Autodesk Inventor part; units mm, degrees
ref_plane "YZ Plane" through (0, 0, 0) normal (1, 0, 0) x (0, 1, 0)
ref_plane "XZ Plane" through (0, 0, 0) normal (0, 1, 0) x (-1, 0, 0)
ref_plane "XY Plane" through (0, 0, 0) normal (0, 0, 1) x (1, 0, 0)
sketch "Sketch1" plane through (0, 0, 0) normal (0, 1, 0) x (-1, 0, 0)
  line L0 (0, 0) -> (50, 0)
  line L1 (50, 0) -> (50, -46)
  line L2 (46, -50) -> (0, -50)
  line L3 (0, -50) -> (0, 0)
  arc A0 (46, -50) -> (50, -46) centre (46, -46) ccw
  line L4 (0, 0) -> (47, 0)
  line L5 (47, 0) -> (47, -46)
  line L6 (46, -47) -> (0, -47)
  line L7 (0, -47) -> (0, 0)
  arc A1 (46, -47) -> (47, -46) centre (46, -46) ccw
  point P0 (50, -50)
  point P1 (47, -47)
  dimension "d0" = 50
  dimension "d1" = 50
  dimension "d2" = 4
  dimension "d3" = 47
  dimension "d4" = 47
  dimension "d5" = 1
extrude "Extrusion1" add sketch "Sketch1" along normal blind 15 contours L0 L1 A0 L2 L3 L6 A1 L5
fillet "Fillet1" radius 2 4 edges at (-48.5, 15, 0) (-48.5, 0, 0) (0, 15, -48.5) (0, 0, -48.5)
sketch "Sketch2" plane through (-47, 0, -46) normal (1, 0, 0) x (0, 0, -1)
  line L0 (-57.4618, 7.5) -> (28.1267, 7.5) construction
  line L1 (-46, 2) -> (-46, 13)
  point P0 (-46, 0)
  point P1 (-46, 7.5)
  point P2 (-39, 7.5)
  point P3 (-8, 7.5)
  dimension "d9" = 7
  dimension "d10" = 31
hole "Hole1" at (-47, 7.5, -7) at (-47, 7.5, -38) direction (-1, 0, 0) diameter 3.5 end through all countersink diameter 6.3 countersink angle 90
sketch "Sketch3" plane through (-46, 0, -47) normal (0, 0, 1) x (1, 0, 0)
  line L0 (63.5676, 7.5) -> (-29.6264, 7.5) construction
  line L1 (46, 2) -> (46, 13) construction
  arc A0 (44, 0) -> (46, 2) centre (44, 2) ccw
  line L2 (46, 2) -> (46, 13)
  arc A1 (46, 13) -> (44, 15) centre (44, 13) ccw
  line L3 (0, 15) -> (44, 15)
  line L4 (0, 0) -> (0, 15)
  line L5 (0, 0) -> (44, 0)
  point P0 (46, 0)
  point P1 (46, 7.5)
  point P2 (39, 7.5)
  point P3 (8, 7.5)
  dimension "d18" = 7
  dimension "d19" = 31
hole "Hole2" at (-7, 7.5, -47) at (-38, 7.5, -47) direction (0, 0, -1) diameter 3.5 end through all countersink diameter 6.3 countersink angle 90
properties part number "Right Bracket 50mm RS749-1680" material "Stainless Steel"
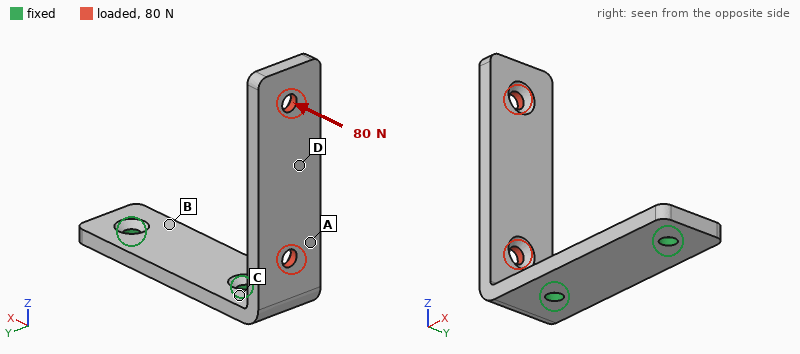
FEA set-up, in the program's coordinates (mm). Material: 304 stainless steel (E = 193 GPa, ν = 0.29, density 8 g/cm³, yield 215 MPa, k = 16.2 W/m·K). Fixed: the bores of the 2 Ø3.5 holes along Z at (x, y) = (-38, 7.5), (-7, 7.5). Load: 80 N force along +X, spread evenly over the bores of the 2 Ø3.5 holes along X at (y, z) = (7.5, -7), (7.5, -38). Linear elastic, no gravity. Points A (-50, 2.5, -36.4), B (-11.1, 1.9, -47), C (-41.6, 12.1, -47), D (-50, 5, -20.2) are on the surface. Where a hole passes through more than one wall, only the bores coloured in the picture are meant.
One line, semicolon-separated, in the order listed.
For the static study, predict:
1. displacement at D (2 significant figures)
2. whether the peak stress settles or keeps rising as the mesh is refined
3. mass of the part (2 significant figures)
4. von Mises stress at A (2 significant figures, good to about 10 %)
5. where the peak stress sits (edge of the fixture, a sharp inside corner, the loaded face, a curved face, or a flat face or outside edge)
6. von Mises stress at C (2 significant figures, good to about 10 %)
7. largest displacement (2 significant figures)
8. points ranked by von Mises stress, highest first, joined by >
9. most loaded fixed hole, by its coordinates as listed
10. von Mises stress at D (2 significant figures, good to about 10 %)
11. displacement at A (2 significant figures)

0.20 mm; keeps rising; 33 g; 66 MPa; edge of the fixture; 98 MPa; 0.39 mm; C > A > D > B; (-7, 7.5); 24 MPa; 0.072 mm
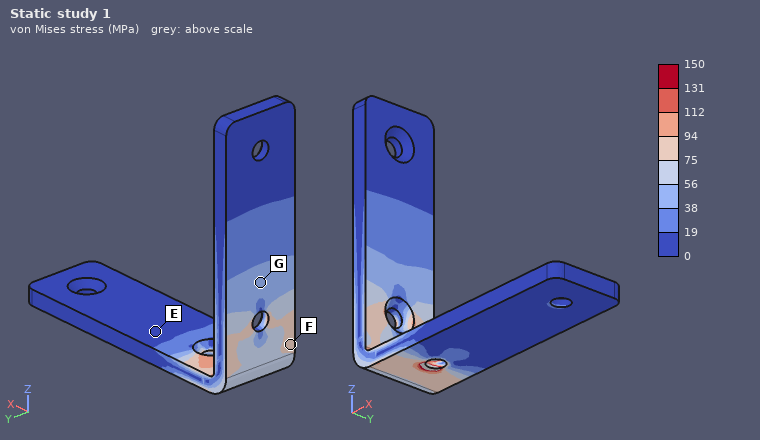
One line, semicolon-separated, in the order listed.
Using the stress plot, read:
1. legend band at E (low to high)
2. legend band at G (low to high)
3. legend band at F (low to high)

0 to 19 MPa; 38 to 56 MPa; 75 to 94 MPa
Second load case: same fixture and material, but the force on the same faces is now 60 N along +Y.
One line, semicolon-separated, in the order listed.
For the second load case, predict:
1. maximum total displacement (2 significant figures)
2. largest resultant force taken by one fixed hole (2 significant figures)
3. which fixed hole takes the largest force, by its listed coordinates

0.10 mm; 71 N; (-38, 7.5)
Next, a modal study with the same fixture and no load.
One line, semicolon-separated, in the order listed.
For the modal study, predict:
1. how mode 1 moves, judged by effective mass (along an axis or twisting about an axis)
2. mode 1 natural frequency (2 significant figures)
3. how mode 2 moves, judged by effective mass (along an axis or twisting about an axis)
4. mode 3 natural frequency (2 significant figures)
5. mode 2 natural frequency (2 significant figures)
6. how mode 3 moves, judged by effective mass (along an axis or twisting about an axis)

along X; 730 Hz; along Y; 4200 Hz; 1200 Hz; along Z
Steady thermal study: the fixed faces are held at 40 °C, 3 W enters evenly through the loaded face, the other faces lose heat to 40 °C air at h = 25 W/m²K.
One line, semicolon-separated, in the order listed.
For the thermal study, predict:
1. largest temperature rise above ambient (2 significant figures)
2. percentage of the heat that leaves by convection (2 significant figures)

63 K; 64 %
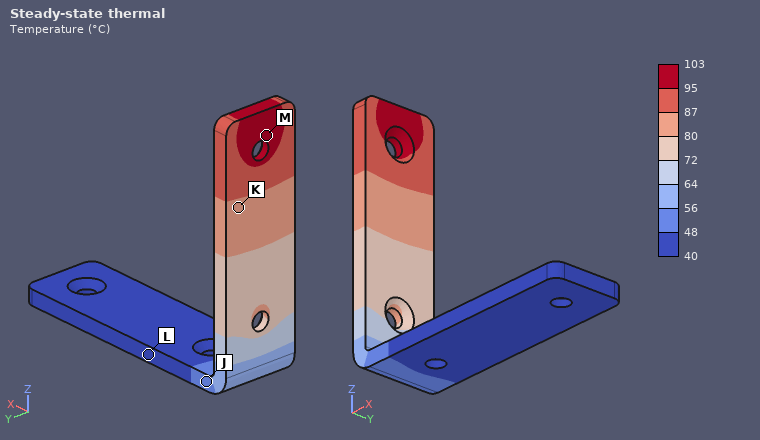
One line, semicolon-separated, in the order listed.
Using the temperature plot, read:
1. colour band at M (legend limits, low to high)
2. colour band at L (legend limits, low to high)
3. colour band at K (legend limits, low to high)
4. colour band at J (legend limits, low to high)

95 to 103 °C; 40 to 48 °C; 80 to 87 °C; 48 to 56 °C
